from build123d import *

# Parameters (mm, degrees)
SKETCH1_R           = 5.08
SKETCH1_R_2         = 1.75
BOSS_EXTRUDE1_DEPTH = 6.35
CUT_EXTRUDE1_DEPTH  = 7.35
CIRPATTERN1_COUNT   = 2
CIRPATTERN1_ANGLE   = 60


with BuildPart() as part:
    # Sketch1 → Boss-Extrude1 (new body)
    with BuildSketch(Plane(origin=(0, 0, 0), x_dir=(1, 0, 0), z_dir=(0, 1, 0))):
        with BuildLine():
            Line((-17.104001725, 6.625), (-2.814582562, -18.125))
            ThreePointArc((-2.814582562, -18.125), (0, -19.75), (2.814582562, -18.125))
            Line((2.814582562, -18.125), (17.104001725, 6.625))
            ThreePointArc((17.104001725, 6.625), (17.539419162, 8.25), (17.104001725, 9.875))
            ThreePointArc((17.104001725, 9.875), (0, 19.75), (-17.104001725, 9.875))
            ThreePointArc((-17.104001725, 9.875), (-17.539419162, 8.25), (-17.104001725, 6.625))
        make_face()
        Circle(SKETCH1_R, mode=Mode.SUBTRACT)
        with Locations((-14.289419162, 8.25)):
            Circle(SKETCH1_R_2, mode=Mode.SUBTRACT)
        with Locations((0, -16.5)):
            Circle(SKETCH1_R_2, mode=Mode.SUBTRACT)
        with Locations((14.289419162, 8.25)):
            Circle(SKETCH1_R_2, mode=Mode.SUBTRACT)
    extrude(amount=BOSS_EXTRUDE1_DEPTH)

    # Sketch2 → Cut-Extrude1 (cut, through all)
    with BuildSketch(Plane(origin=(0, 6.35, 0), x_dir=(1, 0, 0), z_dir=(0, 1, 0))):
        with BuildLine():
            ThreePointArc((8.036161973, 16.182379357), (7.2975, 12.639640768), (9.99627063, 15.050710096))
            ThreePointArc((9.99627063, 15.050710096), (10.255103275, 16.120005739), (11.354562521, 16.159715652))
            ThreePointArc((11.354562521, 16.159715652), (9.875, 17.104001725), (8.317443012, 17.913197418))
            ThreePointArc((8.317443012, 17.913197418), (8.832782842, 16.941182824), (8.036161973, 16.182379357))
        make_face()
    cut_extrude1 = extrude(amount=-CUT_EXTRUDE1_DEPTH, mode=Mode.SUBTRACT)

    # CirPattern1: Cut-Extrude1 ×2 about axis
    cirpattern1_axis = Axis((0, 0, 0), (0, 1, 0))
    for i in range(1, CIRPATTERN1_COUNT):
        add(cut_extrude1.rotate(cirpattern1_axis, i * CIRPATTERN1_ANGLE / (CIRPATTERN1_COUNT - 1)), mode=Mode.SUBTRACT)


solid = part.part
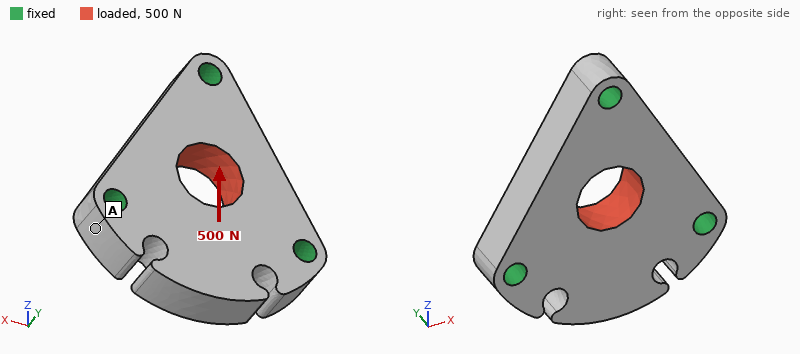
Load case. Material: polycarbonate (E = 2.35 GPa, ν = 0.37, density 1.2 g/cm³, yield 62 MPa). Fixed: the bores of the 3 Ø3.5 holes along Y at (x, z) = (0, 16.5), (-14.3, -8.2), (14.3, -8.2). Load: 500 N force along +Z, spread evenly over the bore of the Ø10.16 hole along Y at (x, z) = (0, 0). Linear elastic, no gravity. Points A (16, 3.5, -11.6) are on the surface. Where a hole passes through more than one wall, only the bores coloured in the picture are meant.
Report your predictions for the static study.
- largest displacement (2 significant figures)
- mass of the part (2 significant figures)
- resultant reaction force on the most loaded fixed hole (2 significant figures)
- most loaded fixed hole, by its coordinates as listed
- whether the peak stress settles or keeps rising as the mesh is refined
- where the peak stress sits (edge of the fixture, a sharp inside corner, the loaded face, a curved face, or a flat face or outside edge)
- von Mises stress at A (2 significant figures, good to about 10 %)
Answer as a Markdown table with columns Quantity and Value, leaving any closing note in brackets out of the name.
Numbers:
| Quantity | Value |
|---|---|
| largest displacement | 37 µm |
| mass of the part | 5.4 g |
| resultant reaction force on the most loaded fixed hole | 210 N |
| most loaded fixed hole, by its coordinates as listed | (0, 16.5) |
| whether the peak stress settles or keeps rising as the mesh is refined | keeps rising |
| where the peak stress sits | edge of the fixture |
| von Mises stress at A | 2.4 MPa |
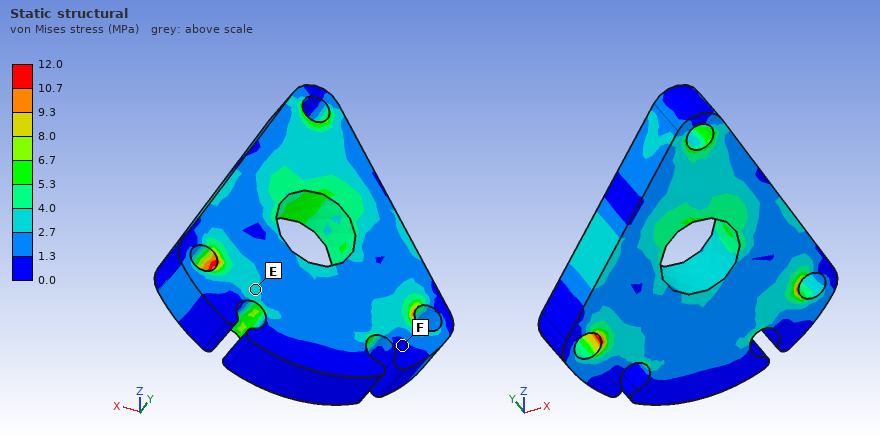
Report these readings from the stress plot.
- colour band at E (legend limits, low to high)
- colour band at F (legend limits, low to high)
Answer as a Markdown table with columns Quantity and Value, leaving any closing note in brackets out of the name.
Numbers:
| Quantity | Value |
|---|---|
| colour band at E | 2.7 to 4.0 MPa |
| colour band at F | 0.0 to 1.3 MPa |
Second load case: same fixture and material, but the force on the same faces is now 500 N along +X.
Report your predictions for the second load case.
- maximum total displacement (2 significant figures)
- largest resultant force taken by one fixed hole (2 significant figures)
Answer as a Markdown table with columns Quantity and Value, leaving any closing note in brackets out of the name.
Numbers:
| Quantity | Value |
|---|---|
| maximum total displacement | 44 µm |
| largest resultant force taken by one fixed hole | 200 N |
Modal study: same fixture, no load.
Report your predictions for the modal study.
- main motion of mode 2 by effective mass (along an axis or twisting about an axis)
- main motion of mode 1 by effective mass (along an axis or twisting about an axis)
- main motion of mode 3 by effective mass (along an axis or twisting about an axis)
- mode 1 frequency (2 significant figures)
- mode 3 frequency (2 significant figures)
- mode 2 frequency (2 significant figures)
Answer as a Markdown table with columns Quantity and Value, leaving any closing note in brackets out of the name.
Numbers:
| Quantity | Value |
|---|---|
| main motion of mode 2 by effective mass | along Y |
| main motion of mode 1 by effective mass | along Y |
| main motion of mode 3 by effective mass | along Z |
| mode 1 frequency | 5300 Hz |
| mode 3 frequency | 10 kHz |
| mode 2 frequency | 8800 Hz |
